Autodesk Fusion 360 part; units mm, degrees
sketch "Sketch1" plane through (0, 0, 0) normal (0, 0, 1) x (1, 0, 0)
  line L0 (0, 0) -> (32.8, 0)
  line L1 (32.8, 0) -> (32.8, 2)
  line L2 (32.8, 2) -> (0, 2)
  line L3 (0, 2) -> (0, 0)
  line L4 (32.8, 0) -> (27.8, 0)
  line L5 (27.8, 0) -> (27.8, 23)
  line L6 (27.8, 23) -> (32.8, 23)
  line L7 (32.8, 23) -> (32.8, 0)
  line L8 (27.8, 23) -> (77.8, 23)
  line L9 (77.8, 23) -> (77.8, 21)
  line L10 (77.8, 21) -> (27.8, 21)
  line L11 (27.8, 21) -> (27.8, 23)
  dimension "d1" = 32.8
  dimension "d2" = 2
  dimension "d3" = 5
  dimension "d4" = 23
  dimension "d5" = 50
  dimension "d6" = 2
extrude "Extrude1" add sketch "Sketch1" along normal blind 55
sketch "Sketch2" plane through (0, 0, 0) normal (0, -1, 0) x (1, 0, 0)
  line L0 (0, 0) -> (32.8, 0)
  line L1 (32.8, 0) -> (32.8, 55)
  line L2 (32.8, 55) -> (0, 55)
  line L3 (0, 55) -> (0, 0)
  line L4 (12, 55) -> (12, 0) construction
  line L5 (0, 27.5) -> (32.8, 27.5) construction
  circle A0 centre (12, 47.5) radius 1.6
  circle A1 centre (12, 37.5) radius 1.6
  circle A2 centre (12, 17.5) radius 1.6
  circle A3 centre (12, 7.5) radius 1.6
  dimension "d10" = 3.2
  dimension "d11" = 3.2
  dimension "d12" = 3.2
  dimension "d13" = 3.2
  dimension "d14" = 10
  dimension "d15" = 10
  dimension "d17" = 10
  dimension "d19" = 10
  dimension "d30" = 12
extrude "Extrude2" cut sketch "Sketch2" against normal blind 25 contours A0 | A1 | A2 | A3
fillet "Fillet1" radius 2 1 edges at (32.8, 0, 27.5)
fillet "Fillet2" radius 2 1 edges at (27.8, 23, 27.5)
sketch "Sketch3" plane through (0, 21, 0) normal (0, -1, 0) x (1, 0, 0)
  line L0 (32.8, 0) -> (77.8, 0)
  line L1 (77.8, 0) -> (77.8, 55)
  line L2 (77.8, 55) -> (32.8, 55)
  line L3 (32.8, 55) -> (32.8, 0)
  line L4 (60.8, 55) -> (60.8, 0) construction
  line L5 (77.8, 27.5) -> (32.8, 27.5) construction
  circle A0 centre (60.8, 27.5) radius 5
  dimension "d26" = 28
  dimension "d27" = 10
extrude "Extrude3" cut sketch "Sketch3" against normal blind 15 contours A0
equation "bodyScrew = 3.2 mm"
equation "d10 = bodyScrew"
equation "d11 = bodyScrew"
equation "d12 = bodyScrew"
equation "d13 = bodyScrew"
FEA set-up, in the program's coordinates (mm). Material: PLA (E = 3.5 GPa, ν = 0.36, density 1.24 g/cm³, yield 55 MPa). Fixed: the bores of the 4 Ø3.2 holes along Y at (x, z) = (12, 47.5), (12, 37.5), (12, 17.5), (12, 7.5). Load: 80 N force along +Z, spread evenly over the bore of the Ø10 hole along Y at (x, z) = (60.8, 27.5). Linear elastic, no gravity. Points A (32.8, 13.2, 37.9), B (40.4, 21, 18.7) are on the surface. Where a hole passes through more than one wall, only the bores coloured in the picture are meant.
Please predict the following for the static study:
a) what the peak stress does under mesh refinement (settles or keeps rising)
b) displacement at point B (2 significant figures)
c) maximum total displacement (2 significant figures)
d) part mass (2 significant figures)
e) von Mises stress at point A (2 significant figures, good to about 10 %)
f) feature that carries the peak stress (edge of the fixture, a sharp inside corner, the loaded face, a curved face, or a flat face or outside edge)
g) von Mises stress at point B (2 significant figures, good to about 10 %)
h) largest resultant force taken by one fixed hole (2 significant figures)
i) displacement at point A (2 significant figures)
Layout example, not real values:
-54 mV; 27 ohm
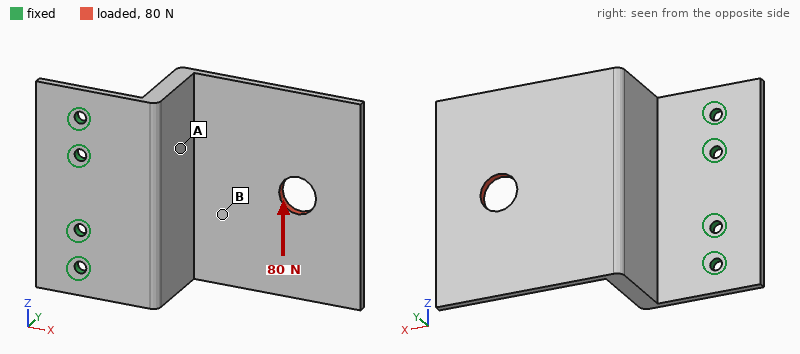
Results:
keeps rising; 0.43 mm; 1.0 mm; 17 g; 7.9 MPa; edge of the fixture; 3.2 MPa; 91 N; 0.23 mm
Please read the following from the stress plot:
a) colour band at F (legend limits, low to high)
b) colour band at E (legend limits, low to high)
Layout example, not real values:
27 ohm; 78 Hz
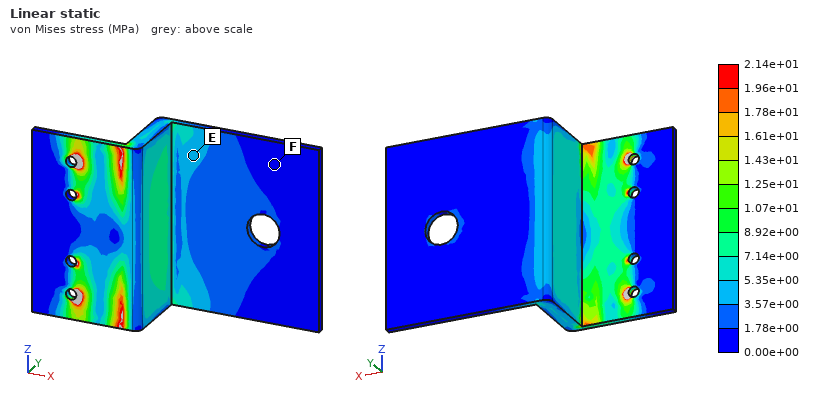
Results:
0.00e+00 to 1.78e+00 MPa; 3.57e+00 to 5.35e+00 MPa
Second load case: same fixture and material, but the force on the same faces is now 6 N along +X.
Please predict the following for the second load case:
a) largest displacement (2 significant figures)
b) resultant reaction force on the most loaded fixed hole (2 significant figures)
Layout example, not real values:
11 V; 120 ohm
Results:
0.92 mm; 2.0 N
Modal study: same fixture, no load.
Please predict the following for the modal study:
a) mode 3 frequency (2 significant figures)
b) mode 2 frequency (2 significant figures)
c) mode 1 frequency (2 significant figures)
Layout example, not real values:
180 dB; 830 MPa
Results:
460 Hz; 440 Hz; 120 Hz
